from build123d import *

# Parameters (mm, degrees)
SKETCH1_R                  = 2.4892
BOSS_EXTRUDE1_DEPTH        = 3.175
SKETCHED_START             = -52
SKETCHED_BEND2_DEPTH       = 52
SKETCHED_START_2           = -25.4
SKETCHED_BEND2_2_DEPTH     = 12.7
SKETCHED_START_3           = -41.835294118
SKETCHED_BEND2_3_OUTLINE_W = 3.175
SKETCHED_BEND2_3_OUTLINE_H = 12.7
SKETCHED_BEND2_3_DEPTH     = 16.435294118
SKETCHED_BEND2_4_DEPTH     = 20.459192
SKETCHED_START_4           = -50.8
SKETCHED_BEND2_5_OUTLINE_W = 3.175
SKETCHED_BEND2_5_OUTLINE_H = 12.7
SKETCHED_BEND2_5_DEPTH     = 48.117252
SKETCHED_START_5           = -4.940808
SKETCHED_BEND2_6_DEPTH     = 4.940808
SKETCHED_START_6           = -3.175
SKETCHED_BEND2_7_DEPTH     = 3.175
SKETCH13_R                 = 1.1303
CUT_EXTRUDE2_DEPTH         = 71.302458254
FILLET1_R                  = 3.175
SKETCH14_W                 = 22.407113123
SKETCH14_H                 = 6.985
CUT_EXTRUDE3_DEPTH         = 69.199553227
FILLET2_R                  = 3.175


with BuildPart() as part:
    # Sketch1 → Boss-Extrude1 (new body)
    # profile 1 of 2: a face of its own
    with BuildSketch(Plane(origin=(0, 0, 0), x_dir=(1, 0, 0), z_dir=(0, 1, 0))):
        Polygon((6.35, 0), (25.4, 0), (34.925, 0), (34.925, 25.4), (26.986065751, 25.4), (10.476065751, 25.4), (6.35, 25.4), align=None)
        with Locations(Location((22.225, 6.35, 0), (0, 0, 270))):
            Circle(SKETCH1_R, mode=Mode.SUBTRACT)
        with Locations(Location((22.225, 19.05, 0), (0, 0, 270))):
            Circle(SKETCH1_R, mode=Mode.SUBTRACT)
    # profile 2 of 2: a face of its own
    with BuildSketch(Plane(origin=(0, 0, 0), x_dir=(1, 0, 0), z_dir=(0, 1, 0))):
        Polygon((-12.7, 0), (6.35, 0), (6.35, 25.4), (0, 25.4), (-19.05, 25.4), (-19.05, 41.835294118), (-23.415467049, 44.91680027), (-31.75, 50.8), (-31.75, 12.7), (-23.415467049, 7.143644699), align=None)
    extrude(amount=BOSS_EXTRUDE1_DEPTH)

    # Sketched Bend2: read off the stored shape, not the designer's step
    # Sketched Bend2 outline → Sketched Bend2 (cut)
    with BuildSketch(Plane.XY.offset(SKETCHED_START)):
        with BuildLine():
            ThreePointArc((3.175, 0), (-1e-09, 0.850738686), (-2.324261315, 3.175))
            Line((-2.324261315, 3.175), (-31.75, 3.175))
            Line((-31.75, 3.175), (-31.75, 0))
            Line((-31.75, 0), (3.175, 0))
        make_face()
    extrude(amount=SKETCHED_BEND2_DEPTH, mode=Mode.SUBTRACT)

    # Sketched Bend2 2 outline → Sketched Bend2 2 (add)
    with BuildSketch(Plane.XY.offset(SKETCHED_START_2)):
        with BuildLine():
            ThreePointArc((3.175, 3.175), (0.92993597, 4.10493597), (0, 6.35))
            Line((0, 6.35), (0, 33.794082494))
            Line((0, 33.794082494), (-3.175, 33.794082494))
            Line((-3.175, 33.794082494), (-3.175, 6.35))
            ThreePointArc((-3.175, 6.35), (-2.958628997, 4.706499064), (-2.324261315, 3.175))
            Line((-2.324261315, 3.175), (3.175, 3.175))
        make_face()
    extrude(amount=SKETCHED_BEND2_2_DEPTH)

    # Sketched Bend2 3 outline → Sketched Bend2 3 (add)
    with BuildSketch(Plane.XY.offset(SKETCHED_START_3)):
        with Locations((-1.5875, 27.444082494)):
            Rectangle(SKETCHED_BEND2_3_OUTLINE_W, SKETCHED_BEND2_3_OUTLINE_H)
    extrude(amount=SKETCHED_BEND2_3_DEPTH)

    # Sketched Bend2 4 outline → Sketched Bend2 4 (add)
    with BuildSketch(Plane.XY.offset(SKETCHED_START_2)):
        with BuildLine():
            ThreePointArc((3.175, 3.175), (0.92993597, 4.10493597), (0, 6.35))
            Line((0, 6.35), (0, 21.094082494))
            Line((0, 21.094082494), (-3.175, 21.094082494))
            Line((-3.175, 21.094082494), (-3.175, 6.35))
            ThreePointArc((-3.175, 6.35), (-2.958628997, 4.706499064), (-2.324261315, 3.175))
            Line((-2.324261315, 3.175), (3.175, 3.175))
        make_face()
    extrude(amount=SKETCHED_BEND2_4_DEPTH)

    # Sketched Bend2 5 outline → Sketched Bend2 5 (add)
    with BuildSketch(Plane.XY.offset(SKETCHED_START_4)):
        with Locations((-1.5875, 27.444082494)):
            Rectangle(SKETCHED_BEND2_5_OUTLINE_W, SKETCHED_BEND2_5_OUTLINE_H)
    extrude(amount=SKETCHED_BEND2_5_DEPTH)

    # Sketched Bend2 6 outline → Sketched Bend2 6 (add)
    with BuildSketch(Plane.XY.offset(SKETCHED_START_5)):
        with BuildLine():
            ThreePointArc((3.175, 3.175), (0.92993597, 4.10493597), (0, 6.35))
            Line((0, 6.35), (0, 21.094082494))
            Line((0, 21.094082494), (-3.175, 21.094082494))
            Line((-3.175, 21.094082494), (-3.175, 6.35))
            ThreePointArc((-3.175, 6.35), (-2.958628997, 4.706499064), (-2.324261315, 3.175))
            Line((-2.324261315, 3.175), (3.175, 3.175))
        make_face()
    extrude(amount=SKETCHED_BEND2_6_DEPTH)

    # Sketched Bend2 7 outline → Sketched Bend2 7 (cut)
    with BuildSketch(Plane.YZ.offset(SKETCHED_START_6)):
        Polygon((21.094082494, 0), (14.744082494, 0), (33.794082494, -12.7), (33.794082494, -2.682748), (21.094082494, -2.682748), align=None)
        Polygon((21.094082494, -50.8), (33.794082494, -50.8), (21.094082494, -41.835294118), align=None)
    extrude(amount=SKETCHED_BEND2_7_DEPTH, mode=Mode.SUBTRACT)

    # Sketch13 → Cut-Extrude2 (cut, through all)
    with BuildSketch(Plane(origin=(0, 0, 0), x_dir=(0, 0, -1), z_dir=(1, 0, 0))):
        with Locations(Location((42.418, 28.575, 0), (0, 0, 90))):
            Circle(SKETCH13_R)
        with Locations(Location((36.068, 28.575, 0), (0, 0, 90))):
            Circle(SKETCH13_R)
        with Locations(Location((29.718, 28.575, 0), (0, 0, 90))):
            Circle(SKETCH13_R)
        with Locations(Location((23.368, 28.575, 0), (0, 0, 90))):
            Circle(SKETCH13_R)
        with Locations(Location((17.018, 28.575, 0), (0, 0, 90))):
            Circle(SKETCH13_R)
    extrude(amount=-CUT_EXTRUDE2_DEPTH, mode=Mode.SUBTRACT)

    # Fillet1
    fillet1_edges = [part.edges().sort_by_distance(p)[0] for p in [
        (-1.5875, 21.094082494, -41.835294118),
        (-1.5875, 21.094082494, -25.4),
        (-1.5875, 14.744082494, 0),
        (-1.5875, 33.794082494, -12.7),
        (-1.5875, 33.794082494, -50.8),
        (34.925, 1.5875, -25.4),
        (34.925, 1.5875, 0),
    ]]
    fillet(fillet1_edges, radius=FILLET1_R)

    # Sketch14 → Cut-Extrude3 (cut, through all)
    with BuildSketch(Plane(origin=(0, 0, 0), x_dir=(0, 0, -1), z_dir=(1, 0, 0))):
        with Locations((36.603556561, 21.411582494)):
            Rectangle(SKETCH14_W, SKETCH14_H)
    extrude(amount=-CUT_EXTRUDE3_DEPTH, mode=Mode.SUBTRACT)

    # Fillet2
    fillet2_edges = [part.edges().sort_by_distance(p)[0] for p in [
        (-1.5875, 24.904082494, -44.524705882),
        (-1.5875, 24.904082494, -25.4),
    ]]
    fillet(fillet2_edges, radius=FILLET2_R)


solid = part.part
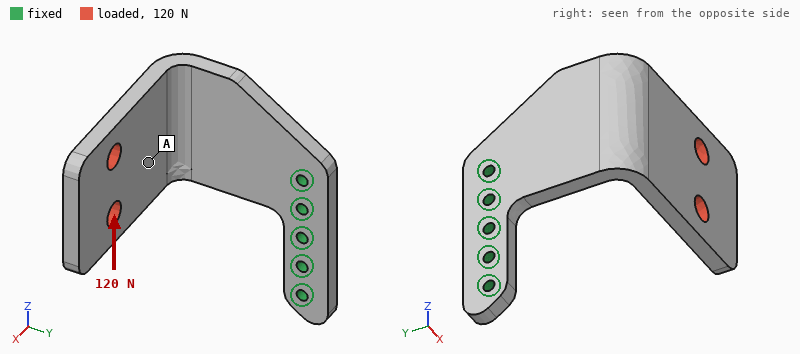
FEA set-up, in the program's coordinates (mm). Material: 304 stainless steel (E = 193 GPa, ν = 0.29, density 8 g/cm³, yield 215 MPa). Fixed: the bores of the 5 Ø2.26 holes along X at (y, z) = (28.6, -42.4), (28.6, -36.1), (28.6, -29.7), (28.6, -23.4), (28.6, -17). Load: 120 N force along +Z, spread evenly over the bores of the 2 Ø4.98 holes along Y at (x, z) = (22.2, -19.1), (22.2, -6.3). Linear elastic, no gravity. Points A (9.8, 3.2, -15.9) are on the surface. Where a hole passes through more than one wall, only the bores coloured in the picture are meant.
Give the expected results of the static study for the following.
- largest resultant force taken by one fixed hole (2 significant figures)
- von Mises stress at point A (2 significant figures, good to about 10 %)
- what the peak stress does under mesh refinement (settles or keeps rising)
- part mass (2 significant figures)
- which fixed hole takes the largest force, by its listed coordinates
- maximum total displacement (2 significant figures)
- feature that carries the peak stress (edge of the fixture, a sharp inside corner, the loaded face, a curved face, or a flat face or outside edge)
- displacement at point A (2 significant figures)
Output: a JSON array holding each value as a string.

["400 N", "11 MPa", "keeps rising", "43 g", "(28.6, -17)", "0.17 mm", "edge of the fixture", "0.053 mm"]
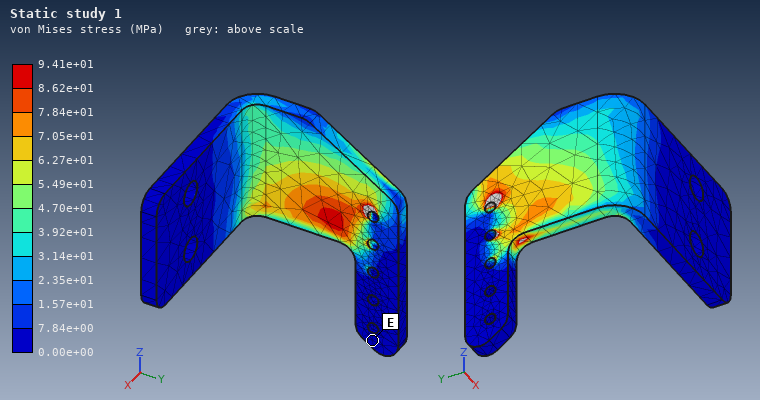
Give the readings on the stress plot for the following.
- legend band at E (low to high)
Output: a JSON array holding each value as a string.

["0.00e+00 to 7.84e+00 MPa"]
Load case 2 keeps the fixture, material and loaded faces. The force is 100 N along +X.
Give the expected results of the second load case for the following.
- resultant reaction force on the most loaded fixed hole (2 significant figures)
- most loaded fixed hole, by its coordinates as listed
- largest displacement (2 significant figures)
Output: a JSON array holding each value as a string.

["110 N", "(28.6, -17)", "0.16 mm"]
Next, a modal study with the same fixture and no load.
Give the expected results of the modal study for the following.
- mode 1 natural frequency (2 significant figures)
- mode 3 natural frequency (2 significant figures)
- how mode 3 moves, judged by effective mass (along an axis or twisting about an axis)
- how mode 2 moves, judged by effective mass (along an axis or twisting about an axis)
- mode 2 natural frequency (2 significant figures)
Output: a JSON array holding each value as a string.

["780 Hz", "2400 Hz", "along X", "along Z", "1200 Hz"]
